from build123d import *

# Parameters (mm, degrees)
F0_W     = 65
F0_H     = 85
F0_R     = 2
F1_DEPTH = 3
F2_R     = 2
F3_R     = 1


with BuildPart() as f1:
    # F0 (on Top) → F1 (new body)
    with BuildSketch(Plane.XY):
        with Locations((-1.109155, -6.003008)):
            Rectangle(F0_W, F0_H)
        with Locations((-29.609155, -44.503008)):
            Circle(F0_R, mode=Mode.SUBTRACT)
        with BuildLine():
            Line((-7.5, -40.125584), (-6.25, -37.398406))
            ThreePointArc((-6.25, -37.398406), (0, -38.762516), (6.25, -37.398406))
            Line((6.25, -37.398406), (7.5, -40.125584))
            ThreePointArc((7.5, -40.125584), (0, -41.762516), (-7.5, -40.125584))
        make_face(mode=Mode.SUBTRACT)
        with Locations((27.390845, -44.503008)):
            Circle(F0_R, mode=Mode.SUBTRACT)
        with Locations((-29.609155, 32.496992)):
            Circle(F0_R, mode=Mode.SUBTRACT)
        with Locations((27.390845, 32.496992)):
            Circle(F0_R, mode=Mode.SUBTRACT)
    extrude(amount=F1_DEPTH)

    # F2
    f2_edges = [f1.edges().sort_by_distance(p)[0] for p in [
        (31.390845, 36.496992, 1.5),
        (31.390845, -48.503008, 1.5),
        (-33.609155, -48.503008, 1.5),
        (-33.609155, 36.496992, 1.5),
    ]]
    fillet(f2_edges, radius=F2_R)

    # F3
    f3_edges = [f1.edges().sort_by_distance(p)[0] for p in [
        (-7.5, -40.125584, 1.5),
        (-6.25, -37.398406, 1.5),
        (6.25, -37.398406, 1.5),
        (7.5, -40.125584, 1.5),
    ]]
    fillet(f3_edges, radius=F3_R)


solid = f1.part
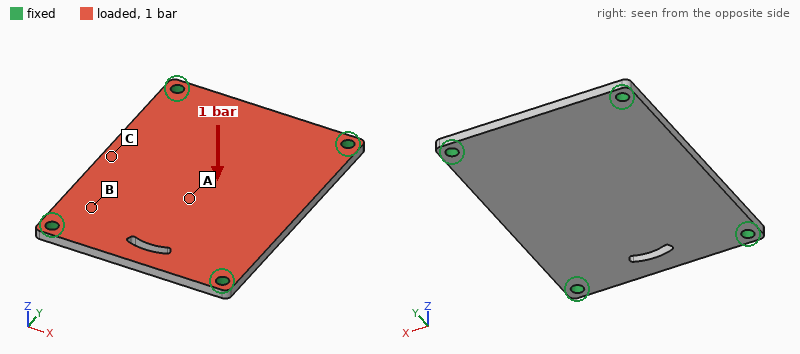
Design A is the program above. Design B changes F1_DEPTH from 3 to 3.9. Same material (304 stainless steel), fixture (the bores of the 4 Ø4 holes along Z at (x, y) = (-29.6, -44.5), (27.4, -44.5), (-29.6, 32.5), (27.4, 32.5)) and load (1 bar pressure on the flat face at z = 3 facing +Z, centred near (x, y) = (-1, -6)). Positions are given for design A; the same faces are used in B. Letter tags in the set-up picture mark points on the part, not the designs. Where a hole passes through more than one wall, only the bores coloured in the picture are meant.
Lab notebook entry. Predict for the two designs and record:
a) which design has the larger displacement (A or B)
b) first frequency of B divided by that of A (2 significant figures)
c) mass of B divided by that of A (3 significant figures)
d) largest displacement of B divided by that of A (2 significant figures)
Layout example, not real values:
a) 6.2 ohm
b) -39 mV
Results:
a) A
b) 1.3
c) 1.30
d) 0.47
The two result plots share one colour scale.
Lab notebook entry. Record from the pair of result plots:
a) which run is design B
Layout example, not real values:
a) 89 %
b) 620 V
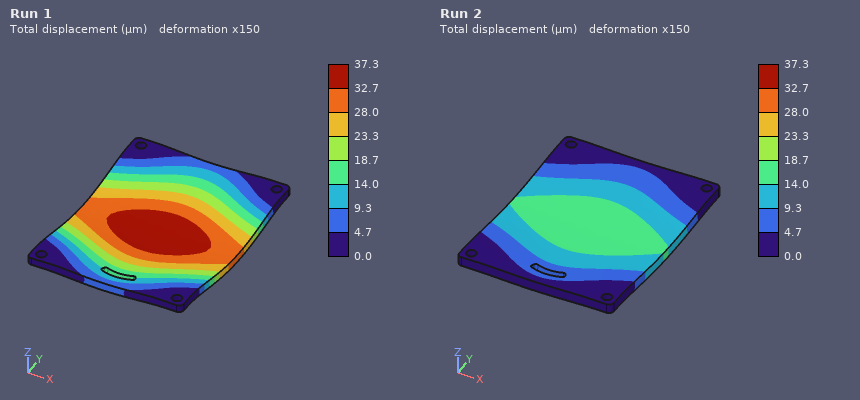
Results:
a) Run 2
